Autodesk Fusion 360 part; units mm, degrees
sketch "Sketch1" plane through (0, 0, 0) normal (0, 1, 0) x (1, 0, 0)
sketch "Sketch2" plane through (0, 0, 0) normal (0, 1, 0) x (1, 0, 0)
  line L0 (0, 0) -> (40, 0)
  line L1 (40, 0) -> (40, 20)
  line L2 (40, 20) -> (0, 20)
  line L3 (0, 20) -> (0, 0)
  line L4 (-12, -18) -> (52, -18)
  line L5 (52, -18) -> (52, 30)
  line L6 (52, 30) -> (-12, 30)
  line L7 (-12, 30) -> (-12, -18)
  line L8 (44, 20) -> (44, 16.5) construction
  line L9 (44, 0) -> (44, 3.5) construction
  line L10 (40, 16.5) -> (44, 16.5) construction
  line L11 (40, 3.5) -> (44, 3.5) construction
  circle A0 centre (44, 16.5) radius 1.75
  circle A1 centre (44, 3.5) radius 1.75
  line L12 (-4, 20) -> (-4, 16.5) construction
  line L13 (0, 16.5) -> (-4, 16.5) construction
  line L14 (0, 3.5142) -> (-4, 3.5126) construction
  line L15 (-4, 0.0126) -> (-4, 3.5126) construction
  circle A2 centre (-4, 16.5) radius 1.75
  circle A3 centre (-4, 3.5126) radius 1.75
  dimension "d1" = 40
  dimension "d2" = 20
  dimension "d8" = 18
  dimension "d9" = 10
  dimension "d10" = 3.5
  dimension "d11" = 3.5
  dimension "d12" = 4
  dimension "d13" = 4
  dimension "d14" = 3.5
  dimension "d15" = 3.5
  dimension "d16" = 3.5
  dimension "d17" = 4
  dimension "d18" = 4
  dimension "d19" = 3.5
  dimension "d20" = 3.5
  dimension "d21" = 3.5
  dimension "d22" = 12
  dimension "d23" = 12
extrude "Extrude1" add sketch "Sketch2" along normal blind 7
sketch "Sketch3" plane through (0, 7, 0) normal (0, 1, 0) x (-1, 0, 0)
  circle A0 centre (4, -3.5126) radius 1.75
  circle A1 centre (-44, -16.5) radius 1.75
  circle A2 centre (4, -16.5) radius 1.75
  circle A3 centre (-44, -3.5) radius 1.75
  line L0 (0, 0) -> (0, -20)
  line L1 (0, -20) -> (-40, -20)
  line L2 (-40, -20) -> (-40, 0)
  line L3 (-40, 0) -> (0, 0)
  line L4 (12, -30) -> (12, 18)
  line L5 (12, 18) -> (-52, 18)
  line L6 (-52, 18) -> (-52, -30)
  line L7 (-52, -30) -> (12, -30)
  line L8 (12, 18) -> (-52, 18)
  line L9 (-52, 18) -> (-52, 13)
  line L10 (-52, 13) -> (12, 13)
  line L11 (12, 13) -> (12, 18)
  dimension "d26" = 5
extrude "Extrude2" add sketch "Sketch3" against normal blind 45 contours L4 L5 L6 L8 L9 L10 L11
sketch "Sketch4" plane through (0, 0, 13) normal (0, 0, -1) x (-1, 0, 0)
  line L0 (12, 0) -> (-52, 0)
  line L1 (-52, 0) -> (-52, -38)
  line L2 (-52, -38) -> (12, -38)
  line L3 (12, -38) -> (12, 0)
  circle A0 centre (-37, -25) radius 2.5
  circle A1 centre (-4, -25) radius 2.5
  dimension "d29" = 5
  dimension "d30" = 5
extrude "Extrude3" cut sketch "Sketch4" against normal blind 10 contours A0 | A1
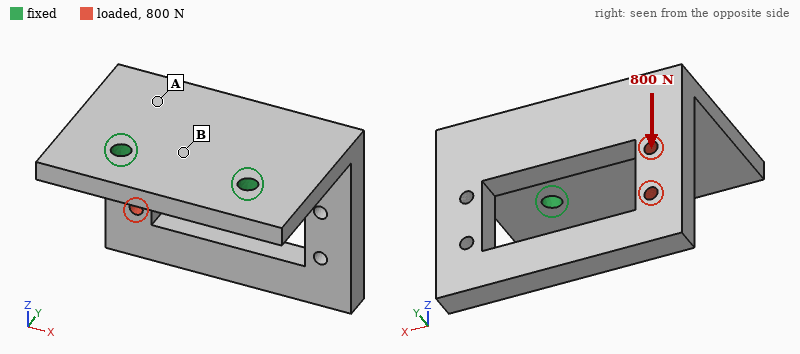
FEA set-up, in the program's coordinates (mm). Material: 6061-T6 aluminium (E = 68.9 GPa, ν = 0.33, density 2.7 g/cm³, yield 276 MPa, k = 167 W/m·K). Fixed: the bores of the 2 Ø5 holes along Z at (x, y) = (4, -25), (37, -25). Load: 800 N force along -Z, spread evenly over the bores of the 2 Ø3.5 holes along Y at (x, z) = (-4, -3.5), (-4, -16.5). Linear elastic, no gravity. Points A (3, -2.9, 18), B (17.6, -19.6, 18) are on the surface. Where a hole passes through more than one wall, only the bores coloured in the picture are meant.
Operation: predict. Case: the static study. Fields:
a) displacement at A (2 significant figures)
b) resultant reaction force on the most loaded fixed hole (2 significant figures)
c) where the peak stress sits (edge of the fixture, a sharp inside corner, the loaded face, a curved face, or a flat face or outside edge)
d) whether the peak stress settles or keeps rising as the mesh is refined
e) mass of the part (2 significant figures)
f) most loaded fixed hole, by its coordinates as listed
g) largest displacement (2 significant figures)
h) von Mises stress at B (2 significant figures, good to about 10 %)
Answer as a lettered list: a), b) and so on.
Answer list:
a) 0.14 mm
b) 880 N
c) edge of the fixture
d) keeps rising
e) 75 g
f) (4, -25)
g) 0.48 mm
h) 52 MPa
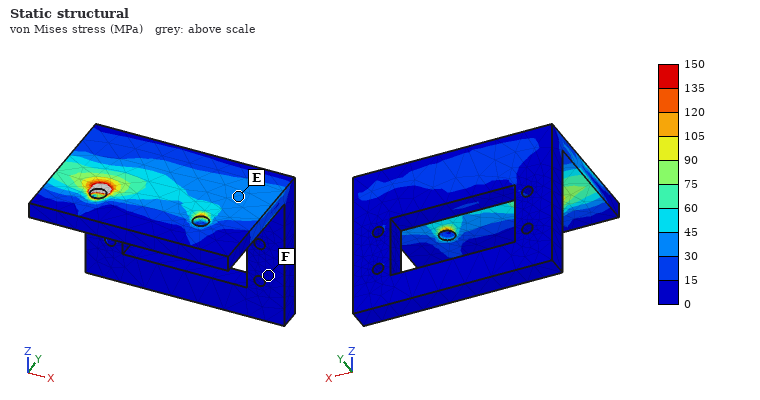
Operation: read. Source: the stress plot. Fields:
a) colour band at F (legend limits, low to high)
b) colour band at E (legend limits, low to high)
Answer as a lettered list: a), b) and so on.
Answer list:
a) 0 to 15 MPa
b) 30 to 45 MPa
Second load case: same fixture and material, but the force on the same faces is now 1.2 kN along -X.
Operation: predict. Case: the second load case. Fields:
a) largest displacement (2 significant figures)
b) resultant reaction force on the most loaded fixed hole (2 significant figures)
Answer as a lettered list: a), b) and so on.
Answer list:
a) 0.29 mm
b) 1.3 kN
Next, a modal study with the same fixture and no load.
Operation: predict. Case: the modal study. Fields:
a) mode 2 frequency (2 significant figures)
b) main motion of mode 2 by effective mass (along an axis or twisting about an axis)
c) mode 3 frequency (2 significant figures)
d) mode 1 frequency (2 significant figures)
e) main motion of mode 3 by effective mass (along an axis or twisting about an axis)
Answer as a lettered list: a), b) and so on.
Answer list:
a) 1800 Hz
b) along X
c) 2900 Hz
d) 980 Hz
e) along Z
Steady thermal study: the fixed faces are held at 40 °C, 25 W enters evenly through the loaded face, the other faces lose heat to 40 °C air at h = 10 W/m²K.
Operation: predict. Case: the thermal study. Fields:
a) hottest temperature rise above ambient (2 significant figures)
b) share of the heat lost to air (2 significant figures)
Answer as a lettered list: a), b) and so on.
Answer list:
a) 44 K
b) 7.3 %
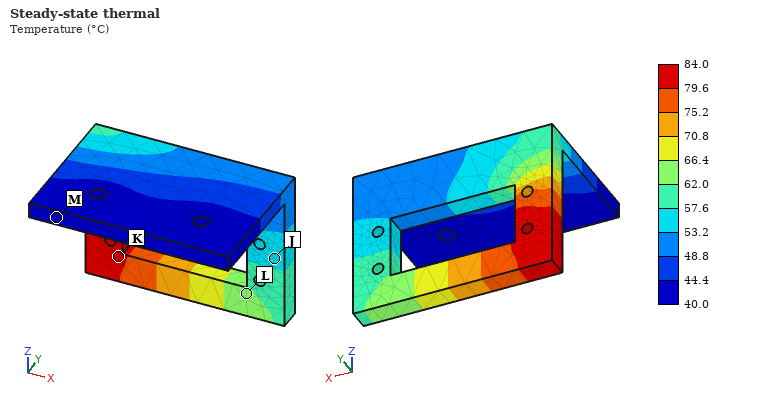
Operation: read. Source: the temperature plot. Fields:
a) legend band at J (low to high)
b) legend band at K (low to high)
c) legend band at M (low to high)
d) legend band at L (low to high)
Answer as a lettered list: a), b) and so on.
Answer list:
a) 53.2 to 57.6 °C
b) 79.6 to 84.0 °C
c) 40.0 to 44.4 °C
d) 62.0 to 66.4 °C
